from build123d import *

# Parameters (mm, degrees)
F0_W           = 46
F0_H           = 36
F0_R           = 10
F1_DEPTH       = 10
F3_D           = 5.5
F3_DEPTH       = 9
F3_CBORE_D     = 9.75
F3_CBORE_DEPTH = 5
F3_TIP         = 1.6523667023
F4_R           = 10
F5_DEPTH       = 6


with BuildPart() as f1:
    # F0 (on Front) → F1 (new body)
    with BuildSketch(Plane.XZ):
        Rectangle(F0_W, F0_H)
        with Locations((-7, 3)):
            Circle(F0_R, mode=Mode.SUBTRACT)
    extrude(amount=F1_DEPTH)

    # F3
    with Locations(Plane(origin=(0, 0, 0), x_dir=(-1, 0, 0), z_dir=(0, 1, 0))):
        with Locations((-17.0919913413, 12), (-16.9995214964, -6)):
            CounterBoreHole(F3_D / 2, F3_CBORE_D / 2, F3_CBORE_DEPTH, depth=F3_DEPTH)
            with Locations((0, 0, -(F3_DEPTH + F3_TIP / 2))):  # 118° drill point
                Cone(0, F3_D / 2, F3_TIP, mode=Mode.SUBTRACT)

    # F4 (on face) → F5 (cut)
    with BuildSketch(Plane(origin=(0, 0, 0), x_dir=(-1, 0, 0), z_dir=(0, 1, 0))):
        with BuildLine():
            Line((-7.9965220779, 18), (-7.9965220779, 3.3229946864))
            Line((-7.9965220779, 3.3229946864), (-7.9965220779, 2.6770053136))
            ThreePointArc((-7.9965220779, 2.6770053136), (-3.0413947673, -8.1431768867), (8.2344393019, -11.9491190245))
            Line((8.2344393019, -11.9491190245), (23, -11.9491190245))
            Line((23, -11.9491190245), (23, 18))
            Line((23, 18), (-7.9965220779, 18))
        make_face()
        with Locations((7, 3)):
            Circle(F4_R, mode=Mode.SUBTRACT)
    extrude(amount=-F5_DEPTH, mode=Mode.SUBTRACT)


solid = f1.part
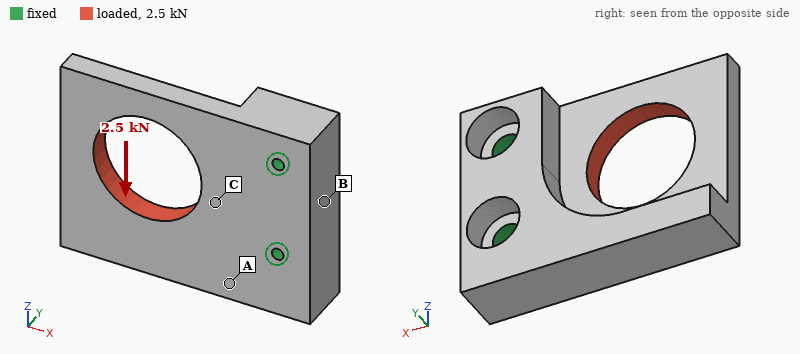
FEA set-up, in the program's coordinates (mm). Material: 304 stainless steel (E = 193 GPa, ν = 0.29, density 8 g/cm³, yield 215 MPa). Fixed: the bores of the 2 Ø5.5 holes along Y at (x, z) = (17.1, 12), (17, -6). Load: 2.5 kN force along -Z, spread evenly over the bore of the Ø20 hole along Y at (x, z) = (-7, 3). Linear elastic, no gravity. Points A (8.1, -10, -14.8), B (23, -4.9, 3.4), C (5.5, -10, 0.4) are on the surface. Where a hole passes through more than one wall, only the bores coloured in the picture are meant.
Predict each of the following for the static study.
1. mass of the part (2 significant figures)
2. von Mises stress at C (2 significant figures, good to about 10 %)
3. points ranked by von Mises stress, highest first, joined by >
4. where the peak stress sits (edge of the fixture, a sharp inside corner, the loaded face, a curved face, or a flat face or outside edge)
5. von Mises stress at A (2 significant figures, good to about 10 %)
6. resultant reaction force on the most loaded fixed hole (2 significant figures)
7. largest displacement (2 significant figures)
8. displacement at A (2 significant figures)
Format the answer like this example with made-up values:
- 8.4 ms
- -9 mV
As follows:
- 72 g
- 67 MPa
- C > A > B
- edge of the fixture
- 35 MPa
- 2.9 kN
- 37 µm
- 6.3 µm
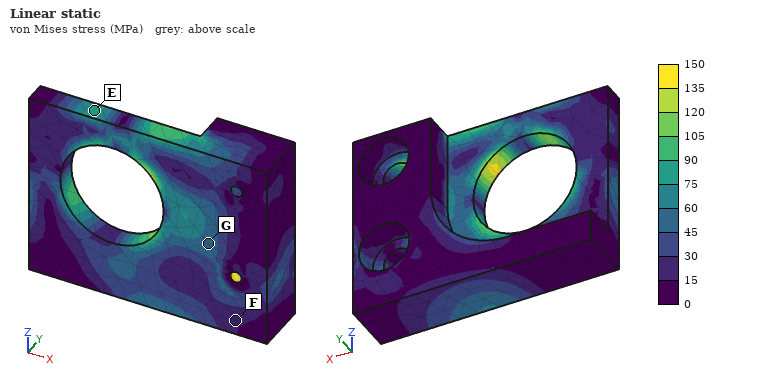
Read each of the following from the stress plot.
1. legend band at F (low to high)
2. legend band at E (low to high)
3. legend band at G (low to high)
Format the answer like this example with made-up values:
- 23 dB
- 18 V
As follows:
- 15 to 30 MPa
- 75 to 90 MPa
- 45 to 60 MPa
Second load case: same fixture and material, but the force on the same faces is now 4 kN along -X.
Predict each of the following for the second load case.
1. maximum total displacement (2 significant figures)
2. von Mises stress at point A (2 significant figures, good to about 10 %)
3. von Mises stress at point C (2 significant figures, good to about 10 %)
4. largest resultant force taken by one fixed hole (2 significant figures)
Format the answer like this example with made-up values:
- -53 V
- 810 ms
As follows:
- 18 µm
- 21 MPa
- 27 MPa
- 2.0 kN
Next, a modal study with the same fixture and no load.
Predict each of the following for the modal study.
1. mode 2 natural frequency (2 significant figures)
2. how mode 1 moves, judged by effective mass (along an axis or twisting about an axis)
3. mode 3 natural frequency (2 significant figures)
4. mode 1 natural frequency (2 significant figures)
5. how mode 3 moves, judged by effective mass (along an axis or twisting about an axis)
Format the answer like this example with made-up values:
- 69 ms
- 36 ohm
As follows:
- 5600 Hz
- along Y
- 8200 Hz
- 3300 Hz
- along Z
